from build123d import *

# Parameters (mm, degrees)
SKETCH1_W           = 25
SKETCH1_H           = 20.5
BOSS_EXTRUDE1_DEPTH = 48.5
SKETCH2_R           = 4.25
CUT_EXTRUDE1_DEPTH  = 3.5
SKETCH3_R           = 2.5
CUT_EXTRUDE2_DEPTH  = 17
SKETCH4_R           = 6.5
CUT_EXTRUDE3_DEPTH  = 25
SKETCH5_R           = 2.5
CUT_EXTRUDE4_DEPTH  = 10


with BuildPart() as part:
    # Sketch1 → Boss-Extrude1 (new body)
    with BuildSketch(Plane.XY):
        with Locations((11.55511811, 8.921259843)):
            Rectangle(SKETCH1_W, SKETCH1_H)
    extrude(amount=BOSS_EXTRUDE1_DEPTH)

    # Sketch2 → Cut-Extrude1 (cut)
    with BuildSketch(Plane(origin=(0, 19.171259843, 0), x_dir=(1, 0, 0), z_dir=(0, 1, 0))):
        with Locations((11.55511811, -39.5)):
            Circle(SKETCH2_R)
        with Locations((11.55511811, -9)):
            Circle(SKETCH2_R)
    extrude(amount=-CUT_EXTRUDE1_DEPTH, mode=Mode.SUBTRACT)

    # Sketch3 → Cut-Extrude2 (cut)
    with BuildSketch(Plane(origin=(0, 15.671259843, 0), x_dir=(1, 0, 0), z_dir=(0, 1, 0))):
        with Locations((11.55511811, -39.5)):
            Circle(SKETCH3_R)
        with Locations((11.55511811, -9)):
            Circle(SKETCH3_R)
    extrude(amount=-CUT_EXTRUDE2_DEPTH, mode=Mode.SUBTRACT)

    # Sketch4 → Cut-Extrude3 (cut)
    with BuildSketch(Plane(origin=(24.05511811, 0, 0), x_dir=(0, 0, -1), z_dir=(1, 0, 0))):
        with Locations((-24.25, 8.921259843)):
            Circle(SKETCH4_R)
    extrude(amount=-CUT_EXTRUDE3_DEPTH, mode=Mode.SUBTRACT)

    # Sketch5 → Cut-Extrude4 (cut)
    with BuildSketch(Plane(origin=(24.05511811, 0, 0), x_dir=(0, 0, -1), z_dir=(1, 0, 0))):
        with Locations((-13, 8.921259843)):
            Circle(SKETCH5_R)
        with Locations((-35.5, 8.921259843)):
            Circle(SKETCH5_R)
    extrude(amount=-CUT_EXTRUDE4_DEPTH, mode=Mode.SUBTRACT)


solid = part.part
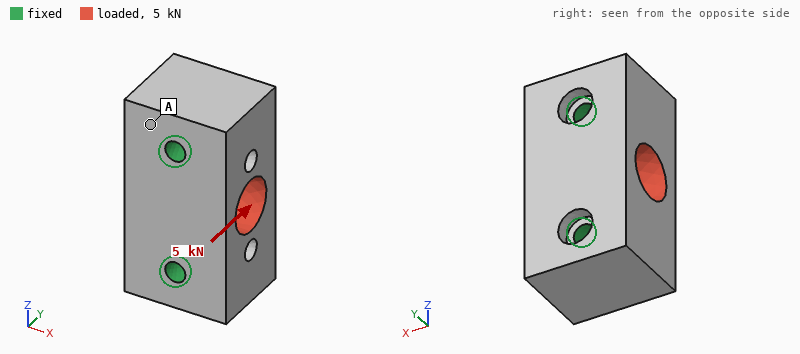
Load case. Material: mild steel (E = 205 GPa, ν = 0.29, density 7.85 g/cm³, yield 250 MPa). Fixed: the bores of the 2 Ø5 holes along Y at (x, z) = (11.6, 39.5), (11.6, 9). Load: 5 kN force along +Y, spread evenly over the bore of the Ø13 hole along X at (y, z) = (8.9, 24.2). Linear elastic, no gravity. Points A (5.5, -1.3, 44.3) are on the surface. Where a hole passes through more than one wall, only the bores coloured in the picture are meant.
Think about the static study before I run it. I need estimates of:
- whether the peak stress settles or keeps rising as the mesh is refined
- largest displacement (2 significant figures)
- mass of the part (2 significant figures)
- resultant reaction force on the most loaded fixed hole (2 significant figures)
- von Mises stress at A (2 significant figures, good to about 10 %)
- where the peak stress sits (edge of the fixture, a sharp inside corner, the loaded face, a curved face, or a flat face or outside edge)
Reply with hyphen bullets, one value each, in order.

- keeps rising
- 2.3 µm
- 160 g
- 2.5 kN
- 5.2 MPa
- edge of the fixture
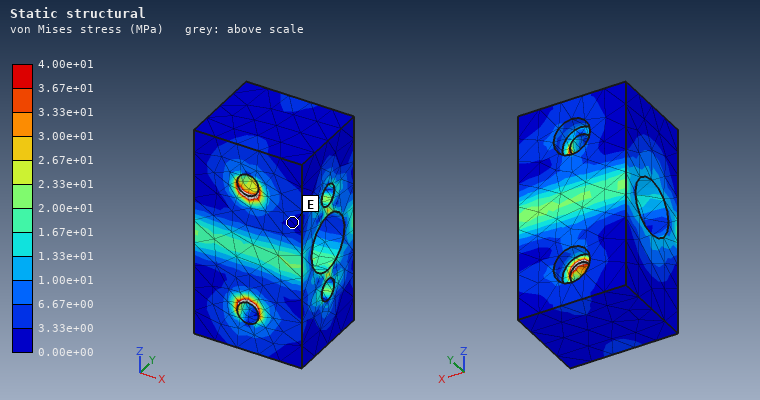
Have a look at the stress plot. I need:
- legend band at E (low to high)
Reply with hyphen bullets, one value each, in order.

- 0.00e+00 to 3.33e+00 MPa
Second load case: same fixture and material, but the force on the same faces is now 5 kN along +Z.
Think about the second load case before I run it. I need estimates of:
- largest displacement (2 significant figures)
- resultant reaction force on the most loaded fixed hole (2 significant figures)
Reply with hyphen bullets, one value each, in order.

- 0.77 µm
- 2.5 kN
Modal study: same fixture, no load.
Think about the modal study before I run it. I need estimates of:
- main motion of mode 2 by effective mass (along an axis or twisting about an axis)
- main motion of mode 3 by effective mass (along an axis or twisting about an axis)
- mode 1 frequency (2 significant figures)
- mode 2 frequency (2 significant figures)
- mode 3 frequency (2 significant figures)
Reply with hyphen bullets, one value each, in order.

- twisting about Z
- twisting about Y
- 31 kHz
- 33 kHz
- 38 kHz
